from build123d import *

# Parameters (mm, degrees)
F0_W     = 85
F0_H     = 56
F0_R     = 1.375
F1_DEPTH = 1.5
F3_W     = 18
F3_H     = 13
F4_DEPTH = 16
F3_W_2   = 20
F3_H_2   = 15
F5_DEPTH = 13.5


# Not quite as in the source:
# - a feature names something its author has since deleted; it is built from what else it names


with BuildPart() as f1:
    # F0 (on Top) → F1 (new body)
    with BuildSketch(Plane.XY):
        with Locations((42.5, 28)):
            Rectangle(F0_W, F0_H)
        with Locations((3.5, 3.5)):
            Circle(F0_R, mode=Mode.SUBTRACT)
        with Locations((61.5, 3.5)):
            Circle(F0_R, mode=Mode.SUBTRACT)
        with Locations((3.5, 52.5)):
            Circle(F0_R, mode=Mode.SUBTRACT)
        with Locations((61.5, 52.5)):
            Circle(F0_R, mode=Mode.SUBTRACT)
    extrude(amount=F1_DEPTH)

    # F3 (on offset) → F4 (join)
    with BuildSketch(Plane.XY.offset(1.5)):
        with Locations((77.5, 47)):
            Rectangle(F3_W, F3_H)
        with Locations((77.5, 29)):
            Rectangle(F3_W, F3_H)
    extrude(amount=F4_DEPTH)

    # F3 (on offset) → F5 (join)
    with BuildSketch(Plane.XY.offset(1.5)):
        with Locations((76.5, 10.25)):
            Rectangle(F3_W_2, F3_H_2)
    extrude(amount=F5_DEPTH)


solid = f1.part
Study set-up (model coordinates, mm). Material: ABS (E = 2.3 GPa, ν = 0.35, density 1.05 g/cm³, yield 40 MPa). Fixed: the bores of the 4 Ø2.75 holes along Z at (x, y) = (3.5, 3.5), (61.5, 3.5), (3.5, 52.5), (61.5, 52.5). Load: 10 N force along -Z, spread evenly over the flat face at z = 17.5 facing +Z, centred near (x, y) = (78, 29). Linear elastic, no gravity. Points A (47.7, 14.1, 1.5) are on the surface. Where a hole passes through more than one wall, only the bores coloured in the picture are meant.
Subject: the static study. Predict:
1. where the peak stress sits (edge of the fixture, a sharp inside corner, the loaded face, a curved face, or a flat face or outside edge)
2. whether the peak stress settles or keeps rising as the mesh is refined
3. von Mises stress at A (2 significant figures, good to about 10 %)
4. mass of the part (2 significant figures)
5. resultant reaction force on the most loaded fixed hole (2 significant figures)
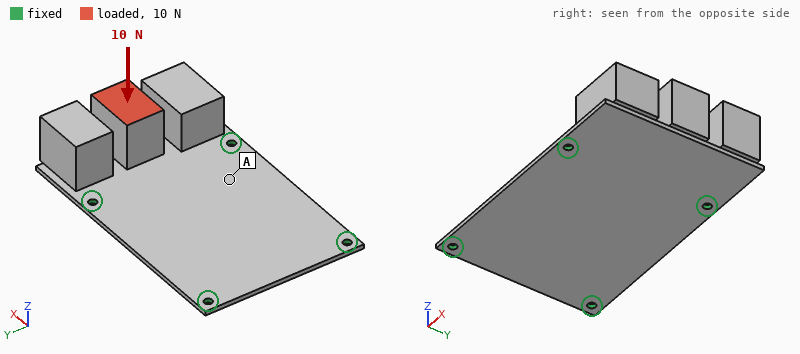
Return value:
edge of the fixture
keeps rising
1.2 MPa
20 g
5.7 N
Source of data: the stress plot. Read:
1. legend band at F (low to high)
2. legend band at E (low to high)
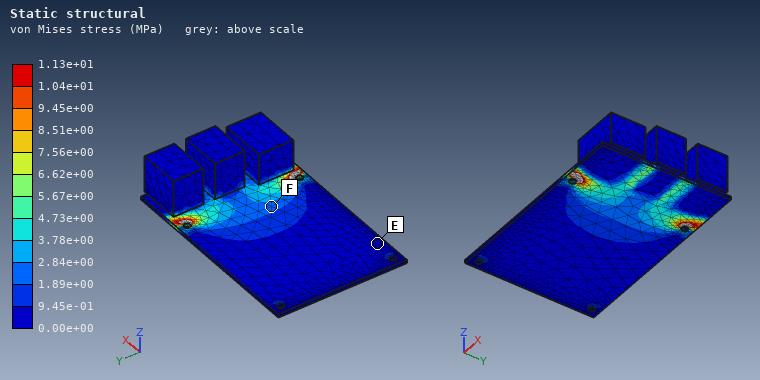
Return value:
1.89e+00 to 2.84e+00 MPa
0.00e+00 to 9.45e-01 MPa
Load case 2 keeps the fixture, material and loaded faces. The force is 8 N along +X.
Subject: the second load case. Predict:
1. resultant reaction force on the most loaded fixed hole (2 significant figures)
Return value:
3.3 N
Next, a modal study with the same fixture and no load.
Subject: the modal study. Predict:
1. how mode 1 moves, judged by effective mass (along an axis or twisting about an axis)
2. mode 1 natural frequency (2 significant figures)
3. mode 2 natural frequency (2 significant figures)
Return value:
along Z
150 Hz
460 Hz
